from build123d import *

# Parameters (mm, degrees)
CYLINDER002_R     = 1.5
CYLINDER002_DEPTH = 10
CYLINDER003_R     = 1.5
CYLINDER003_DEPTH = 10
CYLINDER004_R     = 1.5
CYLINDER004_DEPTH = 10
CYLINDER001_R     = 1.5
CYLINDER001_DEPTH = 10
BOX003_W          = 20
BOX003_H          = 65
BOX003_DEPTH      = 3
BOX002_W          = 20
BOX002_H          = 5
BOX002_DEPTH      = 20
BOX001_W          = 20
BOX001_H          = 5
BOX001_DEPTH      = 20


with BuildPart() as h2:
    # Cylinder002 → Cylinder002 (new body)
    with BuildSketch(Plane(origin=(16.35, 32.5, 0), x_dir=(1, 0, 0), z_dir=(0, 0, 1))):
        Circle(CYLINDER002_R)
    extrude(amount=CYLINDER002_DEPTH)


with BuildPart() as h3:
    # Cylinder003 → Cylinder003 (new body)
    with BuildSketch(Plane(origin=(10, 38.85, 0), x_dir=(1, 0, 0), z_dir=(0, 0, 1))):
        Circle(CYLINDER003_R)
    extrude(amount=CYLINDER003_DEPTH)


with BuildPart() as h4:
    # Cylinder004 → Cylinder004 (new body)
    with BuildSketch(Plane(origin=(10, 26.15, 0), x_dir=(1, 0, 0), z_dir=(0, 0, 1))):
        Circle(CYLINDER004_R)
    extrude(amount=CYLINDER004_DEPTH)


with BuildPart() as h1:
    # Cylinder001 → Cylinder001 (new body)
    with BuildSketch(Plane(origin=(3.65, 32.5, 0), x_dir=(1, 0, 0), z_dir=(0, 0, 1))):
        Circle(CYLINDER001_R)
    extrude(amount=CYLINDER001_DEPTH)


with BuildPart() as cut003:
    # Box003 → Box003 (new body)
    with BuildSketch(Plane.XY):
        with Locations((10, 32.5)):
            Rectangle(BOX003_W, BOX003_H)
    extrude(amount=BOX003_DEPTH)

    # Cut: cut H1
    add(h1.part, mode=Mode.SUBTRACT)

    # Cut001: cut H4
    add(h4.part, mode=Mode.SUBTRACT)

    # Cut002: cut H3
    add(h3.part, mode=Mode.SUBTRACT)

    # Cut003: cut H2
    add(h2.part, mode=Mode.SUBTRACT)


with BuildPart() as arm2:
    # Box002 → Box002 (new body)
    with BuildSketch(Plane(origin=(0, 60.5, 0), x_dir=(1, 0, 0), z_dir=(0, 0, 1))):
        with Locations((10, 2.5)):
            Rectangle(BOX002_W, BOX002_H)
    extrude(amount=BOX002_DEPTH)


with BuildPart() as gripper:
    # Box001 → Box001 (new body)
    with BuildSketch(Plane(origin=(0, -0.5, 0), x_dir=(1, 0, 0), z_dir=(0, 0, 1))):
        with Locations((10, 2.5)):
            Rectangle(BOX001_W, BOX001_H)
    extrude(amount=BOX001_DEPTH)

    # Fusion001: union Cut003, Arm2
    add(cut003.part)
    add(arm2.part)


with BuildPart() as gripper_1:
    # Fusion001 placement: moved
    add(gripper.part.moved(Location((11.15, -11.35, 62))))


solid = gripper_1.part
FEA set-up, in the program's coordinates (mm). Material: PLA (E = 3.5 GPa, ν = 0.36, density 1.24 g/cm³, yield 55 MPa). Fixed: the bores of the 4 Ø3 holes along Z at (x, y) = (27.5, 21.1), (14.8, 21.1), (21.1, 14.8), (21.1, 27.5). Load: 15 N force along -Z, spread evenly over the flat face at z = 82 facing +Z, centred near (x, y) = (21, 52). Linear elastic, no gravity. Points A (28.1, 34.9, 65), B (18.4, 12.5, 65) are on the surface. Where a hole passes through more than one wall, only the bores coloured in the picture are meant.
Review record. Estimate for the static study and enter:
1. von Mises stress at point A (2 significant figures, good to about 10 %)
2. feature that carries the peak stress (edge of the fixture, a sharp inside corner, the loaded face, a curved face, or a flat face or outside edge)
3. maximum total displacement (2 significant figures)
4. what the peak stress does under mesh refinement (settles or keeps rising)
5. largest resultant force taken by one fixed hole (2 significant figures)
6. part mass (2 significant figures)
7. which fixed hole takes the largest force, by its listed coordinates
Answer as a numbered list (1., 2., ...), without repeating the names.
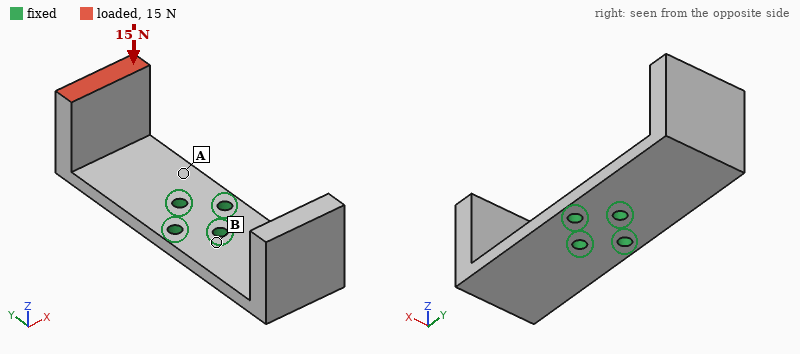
1. 7.8 MPa
2. edge of the fixture
3. 0.70 mm
4. keeps rising
5. 39 N
6. 9.0 g
7. (21.1, 27.5)
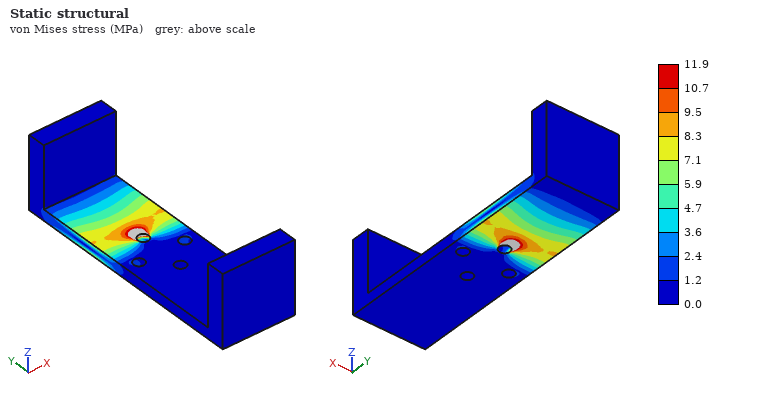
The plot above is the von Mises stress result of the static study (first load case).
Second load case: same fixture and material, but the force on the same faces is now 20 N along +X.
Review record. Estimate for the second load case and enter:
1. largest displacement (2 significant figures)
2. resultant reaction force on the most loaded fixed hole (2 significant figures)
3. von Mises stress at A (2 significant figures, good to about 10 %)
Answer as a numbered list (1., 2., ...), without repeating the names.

1. 0.71 mm
2. 28 N
3. 9.5 MPa
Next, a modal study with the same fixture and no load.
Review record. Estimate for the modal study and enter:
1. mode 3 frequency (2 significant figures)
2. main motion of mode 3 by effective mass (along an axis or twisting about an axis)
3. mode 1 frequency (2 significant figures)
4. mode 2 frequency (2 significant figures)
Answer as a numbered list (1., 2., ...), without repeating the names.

1. 870 Hz
2. twisting about Z
3. 480 Hz
4. 480 Hz
